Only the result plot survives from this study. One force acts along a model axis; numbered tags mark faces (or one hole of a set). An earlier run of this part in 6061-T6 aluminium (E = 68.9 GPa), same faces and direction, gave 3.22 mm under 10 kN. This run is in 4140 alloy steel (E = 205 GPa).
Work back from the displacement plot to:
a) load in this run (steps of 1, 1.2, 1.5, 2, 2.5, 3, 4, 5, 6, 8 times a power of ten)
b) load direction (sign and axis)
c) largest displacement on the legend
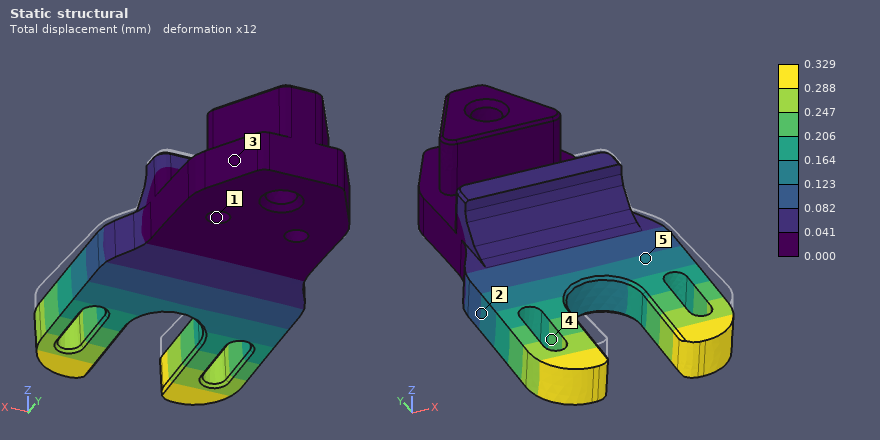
3 kN
-Z
0.329 mm
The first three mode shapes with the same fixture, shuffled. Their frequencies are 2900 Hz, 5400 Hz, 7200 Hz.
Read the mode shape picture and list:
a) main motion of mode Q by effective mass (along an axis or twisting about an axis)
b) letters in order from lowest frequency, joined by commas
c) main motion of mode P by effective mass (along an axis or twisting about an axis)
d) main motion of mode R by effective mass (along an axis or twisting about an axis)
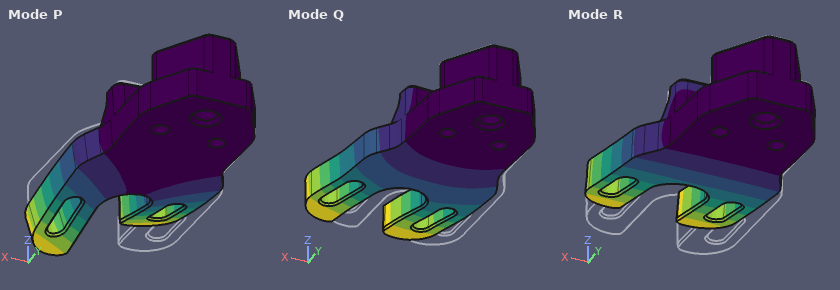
along X
R, P, Q
twisting about Y
along Z
